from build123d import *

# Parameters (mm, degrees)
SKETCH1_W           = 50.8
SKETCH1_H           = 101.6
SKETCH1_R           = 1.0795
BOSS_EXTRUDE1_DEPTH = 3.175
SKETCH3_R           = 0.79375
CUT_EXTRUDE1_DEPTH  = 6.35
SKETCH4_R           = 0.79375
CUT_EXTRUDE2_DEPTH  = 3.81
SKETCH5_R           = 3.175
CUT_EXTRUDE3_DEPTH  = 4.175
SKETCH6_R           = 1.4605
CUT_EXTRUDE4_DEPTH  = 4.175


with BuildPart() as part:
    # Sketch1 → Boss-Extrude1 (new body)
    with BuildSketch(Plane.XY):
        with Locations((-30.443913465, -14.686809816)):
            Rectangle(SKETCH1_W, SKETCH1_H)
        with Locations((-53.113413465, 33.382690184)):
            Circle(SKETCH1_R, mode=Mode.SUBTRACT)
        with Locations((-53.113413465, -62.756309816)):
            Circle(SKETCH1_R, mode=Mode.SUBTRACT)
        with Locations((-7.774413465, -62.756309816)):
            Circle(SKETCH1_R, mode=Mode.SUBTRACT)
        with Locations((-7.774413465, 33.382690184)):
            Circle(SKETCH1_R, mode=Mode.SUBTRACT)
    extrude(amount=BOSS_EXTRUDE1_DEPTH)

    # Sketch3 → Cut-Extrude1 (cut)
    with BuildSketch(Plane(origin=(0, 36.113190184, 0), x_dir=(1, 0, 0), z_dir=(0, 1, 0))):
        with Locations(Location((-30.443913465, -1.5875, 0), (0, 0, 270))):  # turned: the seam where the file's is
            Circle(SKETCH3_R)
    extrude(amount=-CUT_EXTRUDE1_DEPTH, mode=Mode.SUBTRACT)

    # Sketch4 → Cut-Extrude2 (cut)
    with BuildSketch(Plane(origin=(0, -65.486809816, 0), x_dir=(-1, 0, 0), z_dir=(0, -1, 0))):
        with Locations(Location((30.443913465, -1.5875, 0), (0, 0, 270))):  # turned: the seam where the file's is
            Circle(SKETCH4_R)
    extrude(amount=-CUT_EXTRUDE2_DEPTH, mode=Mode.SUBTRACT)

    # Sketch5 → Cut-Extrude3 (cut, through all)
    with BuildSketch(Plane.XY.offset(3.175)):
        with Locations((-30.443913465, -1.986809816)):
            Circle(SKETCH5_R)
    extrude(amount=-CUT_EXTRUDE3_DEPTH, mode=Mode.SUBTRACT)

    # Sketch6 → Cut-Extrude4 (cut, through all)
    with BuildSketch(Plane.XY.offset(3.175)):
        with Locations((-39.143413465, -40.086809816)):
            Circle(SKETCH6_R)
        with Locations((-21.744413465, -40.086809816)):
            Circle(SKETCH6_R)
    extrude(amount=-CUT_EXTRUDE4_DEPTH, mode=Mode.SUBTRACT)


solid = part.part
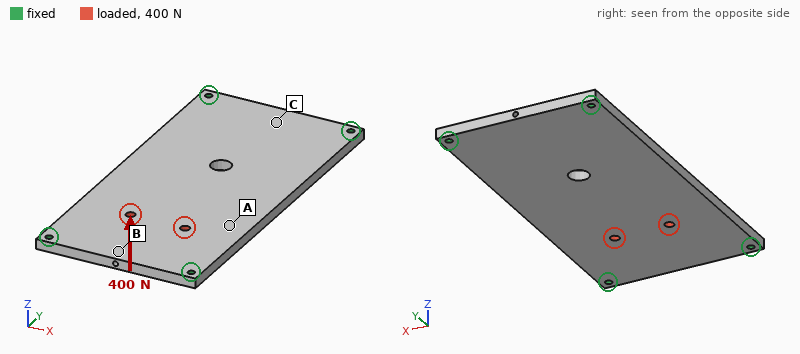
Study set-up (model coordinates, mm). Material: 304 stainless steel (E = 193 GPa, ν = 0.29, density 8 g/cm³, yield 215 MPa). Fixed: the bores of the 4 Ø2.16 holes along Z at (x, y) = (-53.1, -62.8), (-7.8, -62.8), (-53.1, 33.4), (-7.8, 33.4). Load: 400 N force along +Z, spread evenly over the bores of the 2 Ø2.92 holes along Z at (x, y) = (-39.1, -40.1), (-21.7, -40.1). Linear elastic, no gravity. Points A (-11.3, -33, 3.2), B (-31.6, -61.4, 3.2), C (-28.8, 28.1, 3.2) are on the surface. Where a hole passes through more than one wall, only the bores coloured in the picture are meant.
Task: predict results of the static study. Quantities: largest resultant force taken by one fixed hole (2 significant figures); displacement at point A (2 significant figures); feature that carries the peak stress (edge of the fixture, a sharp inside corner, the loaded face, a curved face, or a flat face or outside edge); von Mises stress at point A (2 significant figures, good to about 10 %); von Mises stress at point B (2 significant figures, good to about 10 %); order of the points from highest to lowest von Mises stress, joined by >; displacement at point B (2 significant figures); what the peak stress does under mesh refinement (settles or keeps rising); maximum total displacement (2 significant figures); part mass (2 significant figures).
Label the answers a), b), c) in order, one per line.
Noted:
a) 160 N
b) 55 µm
c) edge of the fixture
d) 35 MPa
e) 18 MPa
f) A > B > C
g) 10 µm
h) keeps rising
i) 63 µm
j) 130 g
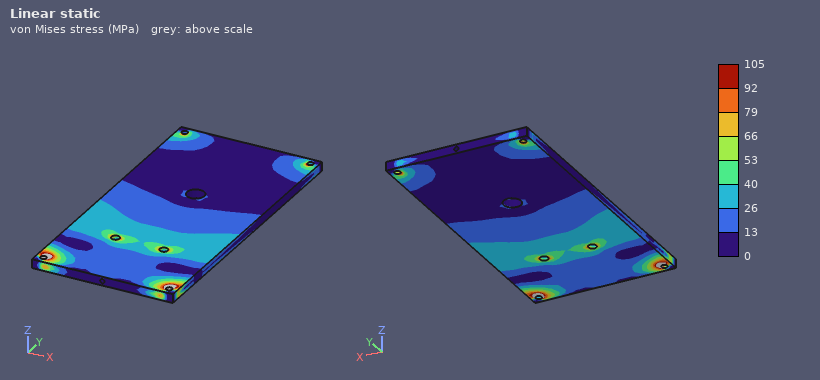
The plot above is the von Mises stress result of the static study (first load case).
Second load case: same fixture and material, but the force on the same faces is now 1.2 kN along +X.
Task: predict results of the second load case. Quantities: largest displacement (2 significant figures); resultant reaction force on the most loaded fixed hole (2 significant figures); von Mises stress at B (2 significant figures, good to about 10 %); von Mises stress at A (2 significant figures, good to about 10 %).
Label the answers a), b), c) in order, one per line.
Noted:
a) 3.3 µm
b) 560 N
c) 5.6 MPa
d) 4.9 MPa
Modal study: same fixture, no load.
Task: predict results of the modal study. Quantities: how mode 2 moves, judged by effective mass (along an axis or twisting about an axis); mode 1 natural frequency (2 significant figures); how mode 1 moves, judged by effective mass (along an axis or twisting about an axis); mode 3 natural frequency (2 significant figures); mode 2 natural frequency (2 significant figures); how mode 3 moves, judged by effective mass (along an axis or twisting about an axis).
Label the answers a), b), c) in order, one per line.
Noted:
a) twisting about Y
b) 1400 Hz
c) along Z
d) 3800 Hz
e) 2700 Hz
f) twisting about X
